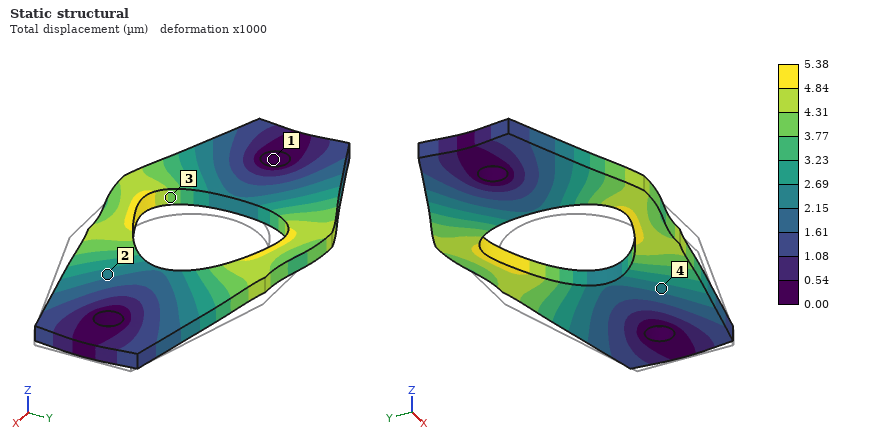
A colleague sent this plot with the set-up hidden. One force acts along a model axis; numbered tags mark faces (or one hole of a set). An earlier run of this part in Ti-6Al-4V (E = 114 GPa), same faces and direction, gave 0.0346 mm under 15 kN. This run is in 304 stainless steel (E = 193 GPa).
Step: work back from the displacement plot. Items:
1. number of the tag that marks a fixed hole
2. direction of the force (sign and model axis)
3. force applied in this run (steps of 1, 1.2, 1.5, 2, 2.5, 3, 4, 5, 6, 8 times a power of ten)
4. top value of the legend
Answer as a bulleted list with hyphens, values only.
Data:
- 1
- -X
- 4 kN
- 5.38 µm
